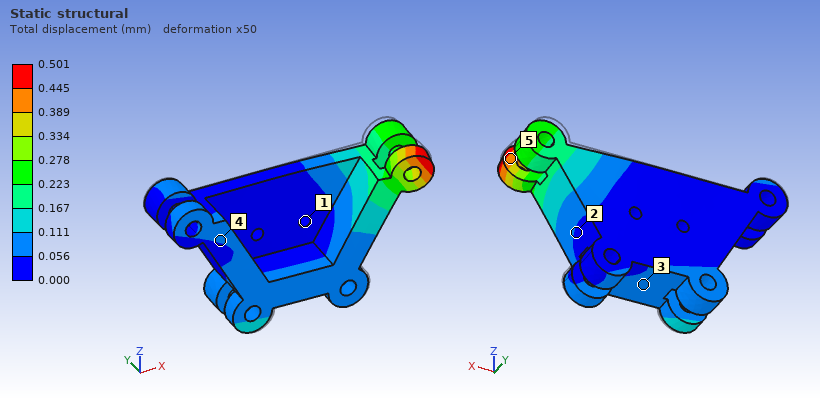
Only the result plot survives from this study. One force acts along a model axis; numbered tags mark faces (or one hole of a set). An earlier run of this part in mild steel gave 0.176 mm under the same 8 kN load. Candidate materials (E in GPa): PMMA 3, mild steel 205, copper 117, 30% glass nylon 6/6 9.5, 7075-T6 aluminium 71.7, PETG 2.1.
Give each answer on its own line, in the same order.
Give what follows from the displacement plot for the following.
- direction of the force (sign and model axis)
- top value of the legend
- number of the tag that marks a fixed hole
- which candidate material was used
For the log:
-Y
0.501 mm
1
7075-T6 aluminium
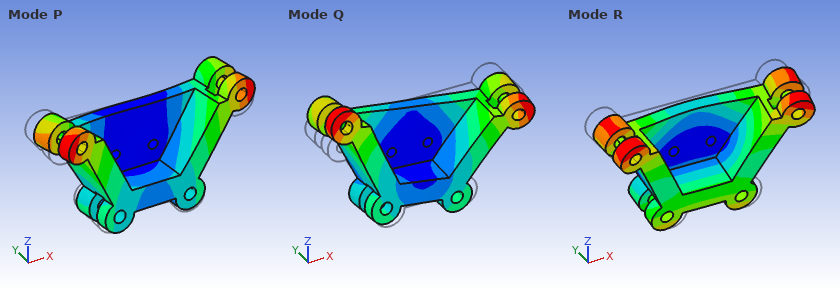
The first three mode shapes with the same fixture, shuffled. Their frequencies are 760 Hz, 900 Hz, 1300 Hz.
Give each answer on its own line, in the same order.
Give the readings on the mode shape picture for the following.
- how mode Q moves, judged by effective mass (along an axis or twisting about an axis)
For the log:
twisting about Y
